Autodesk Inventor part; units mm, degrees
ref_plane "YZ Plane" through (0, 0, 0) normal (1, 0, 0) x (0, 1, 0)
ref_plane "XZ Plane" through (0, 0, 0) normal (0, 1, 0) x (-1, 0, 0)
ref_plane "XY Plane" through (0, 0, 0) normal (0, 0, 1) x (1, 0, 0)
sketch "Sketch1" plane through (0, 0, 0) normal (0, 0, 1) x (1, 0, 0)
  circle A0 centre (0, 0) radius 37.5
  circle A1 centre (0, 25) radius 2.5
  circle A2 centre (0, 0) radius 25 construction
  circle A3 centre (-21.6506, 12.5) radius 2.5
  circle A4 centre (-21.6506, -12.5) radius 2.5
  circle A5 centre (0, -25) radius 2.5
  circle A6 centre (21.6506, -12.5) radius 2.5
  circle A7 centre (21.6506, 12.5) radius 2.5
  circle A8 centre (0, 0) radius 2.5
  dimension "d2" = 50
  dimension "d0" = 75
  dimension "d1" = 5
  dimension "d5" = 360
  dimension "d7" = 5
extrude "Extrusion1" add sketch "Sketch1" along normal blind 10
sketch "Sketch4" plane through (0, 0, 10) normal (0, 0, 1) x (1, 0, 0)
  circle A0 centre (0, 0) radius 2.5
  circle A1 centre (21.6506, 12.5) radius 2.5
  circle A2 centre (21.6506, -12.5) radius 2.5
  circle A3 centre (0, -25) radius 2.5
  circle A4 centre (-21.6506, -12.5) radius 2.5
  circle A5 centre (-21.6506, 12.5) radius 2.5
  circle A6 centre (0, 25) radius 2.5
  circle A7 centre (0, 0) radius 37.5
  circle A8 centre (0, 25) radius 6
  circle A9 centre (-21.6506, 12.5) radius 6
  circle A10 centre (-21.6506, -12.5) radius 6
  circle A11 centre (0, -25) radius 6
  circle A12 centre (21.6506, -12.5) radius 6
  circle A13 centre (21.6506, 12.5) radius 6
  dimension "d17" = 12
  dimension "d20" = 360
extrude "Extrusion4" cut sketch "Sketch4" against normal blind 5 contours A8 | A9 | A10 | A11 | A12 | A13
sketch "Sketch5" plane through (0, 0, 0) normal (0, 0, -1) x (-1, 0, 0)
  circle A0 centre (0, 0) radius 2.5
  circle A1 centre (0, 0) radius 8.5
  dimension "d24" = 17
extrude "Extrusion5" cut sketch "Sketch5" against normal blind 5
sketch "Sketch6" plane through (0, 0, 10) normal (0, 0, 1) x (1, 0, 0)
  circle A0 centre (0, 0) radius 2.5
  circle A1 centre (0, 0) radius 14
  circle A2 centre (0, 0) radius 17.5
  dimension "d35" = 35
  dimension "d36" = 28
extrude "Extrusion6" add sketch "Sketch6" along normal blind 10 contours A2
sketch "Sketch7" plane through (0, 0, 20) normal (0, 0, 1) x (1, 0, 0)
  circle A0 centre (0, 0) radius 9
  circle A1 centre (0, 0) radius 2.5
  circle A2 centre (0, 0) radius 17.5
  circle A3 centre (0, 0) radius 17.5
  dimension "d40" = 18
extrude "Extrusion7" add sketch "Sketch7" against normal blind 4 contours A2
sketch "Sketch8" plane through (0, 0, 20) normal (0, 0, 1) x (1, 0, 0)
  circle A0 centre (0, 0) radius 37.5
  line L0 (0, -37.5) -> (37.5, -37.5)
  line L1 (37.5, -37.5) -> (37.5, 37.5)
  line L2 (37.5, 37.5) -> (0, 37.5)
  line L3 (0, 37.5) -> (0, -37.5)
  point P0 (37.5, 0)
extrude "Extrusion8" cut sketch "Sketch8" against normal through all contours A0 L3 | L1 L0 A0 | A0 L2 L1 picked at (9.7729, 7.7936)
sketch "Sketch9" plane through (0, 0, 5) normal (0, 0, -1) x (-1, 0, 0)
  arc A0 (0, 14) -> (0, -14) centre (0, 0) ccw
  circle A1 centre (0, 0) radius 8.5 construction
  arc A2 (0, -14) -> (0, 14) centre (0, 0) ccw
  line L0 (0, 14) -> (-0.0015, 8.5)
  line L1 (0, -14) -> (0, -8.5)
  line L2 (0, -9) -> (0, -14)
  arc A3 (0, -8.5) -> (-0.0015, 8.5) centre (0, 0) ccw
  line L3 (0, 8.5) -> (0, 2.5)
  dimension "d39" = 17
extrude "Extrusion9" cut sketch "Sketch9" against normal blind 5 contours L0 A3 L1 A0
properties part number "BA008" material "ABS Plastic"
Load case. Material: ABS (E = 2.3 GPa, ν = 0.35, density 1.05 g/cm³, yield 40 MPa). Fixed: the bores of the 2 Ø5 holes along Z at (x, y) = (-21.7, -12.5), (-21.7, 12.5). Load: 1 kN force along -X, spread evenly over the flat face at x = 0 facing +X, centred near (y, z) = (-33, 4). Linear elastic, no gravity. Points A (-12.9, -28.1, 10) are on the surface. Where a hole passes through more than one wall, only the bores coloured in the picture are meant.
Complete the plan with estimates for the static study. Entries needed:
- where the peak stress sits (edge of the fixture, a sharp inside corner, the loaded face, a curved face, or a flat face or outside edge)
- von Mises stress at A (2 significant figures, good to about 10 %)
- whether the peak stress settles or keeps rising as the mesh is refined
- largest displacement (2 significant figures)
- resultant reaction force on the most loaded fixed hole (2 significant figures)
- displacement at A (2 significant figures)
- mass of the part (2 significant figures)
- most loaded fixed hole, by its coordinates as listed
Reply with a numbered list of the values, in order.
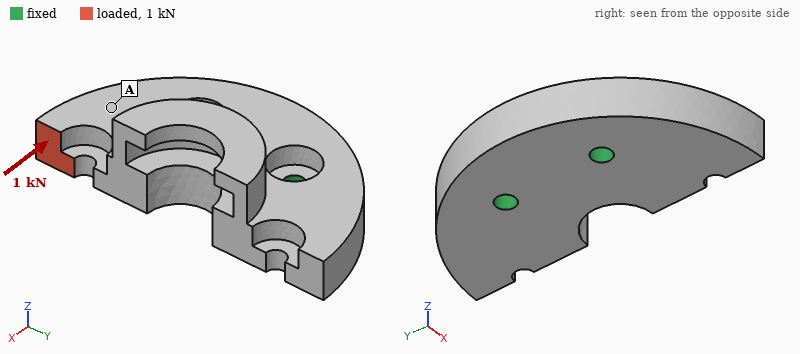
1. edge of the fixture
2. 8.2 MPa
3. keeps rising
4. 0.76 mm
5. 1.7 kN
6. 0.37 mm
7. 22 g
8. (-21.7, -12.5)
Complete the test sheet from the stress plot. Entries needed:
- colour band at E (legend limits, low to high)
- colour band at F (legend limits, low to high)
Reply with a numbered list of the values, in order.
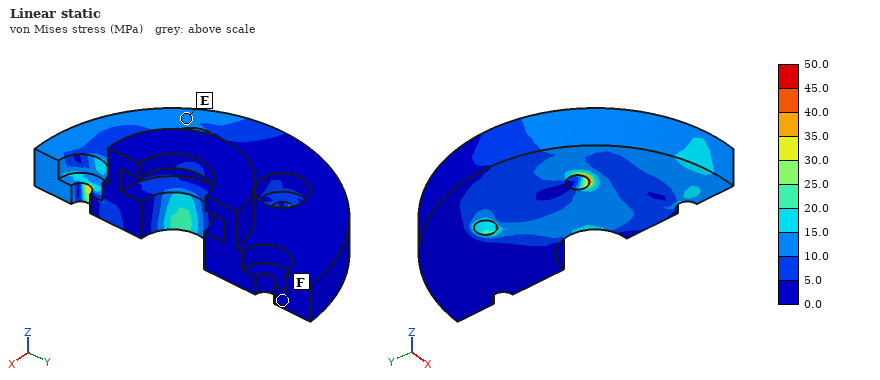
1. 10.0 to 15.0 MPa
2. 0.0 to 5.0 MPa
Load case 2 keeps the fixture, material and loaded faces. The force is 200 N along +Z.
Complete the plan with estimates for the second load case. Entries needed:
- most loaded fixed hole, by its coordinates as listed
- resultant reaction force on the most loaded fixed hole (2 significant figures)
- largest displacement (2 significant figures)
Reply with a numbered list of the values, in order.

1. (-21.7, -12.5)
2. 340 N
3. 0.88 mm
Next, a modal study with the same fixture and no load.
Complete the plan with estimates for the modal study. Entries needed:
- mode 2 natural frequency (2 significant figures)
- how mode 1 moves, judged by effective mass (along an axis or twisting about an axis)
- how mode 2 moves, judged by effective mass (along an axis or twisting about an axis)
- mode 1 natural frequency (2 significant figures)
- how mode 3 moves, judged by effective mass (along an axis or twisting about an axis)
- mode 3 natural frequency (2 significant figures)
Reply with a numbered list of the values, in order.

1. 2300 Hz
2. along Z
3. twisting about X
4. 1700 Hz
5. along Y
6. 3500 Hz
